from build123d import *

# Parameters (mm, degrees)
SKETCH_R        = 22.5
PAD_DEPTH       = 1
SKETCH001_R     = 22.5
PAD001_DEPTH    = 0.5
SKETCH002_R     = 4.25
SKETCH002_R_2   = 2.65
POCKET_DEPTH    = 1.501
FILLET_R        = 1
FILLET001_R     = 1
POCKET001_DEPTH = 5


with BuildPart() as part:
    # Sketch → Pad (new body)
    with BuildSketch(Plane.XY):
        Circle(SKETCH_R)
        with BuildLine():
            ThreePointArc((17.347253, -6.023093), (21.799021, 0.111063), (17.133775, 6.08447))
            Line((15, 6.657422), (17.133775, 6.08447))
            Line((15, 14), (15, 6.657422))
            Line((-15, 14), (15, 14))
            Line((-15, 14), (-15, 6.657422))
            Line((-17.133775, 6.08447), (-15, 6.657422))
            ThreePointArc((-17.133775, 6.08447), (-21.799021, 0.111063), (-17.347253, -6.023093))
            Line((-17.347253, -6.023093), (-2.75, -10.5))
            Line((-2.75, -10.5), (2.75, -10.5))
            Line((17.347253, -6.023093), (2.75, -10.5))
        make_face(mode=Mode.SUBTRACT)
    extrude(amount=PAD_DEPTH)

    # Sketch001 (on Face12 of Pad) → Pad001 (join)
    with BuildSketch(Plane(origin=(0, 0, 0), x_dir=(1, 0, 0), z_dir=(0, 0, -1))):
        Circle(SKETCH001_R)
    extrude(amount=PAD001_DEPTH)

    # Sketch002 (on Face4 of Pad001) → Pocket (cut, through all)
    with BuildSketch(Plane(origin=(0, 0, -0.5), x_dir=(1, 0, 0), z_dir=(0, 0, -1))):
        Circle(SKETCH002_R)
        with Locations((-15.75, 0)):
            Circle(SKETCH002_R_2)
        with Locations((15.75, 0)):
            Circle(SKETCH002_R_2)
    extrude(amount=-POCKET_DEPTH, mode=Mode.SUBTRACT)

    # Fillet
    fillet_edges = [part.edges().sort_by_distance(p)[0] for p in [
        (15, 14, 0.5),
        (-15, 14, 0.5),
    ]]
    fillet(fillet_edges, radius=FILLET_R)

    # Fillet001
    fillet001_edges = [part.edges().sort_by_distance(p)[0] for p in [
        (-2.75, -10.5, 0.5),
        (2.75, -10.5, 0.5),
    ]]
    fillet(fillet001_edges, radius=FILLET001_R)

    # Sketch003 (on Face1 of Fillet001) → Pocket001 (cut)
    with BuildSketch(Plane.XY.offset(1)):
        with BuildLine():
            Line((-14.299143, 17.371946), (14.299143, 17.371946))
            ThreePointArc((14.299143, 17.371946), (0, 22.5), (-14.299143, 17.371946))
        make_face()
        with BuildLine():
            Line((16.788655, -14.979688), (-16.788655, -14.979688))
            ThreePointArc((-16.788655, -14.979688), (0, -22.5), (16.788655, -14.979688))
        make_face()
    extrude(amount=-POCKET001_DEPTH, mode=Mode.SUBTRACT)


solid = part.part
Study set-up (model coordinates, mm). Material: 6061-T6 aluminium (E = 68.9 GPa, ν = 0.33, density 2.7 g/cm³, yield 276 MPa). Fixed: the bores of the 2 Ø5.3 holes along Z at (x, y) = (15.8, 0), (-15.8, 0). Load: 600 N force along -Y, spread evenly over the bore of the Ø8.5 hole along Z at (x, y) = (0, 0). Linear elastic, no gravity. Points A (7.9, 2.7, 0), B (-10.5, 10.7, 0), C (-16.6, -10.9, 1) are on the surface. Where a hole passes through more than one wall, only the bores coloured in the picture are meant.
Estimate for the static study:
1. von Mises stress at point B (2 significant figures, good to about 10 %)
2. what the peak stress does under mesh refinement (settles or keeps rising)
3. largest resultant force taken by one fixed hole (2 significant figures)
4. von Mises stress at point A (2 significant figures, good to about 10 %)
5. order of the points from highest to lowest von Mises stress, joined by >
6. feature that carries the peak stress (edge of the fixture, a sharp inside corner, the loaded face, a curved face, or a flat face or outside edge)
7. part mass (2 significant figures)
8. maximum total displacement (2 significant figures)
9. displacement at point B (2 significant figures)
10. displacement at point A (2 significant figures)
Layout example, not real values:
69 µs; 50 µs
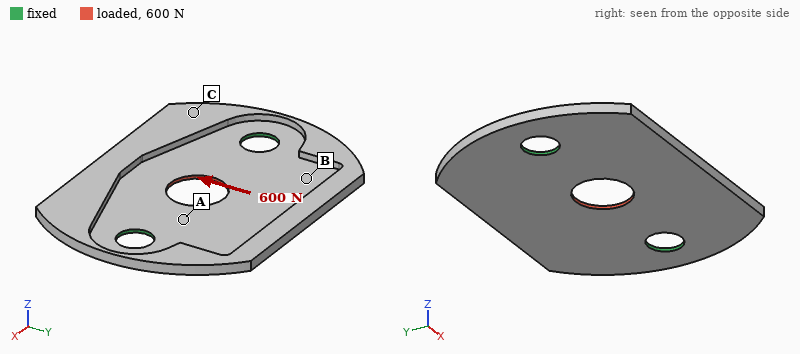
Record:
31 MPa; keeps rising; 300 N; 47 MPa; A > B > C; edge of the fixture; 3.0 g; 31 µm; 6.0 µm; 8.2 µm
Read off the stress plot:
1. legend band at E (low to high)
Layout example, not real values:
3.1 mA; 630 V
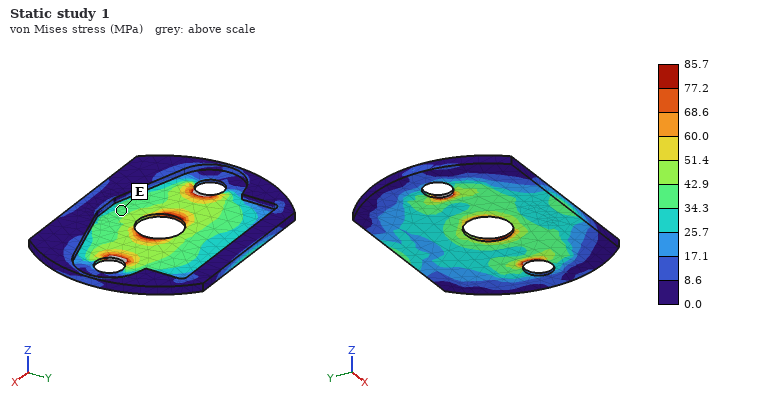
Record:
34.3 to 42.9 MPa
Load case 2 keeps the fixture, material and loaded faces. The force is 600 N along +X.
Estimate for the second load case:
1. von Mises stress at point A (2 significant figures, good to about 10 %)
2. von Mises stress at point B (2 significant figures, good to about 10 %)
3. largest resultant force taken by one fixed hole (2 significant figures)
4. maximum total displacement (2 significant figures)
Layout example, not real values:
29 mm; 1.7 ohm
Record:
48 MPa; 6.9 MPa; 300 N; 9.1 µm
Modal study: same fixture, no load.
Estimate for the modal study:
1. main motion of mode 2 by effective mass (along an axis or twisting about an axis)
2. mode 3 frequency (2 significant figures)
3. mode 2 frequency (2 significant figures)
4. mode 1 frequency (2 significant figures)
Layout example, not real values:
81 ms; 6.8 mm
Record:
along Z; 3600 Hz; 2100 Hz; 1700 Hz
